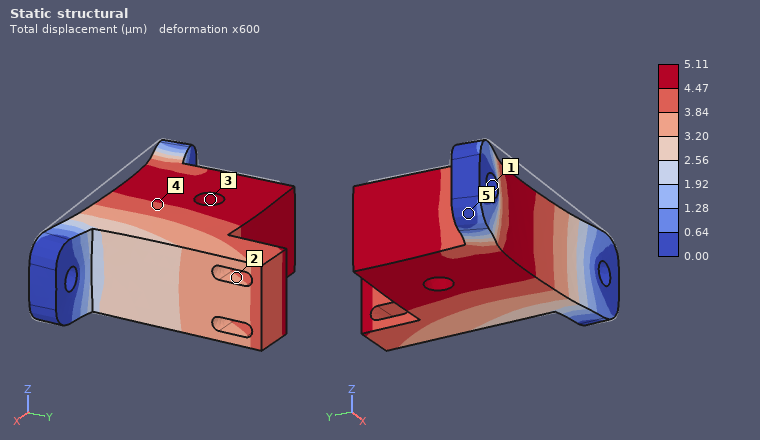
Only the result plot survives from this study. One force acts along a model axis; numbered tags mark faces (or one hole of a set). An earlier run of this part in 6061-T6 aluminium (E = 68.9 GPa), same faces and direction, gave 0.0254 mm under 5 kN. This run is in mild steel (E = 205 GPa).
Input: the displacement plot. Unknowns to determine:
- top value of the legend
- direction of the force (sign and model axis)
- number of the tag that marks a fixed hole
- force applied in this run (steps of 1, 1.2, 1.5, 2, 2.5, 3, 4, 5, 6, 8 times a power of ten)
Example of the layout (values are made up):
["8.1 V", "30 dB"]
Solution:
["5.11 µm", "+Y", "1", "3 kN"]
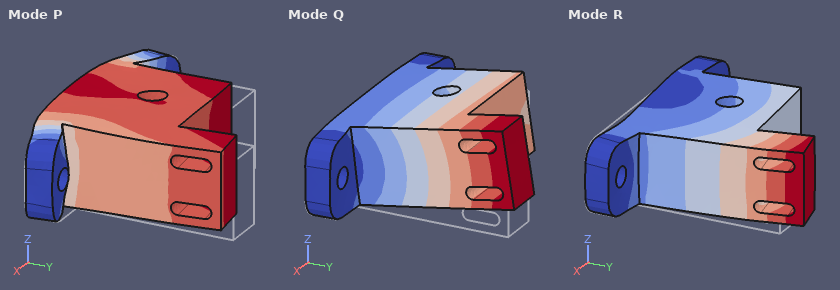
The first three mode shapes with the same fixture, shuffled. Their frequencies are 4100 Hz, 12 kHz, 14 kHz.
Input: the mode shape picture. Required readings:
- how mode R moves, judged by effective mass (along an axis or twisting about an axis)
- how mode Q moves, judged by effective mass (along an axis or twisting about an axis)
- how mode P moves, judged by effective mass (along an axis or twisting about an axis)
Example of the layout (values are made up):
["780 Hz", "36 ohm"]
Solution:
["along X", "along Z", "along Y"]
